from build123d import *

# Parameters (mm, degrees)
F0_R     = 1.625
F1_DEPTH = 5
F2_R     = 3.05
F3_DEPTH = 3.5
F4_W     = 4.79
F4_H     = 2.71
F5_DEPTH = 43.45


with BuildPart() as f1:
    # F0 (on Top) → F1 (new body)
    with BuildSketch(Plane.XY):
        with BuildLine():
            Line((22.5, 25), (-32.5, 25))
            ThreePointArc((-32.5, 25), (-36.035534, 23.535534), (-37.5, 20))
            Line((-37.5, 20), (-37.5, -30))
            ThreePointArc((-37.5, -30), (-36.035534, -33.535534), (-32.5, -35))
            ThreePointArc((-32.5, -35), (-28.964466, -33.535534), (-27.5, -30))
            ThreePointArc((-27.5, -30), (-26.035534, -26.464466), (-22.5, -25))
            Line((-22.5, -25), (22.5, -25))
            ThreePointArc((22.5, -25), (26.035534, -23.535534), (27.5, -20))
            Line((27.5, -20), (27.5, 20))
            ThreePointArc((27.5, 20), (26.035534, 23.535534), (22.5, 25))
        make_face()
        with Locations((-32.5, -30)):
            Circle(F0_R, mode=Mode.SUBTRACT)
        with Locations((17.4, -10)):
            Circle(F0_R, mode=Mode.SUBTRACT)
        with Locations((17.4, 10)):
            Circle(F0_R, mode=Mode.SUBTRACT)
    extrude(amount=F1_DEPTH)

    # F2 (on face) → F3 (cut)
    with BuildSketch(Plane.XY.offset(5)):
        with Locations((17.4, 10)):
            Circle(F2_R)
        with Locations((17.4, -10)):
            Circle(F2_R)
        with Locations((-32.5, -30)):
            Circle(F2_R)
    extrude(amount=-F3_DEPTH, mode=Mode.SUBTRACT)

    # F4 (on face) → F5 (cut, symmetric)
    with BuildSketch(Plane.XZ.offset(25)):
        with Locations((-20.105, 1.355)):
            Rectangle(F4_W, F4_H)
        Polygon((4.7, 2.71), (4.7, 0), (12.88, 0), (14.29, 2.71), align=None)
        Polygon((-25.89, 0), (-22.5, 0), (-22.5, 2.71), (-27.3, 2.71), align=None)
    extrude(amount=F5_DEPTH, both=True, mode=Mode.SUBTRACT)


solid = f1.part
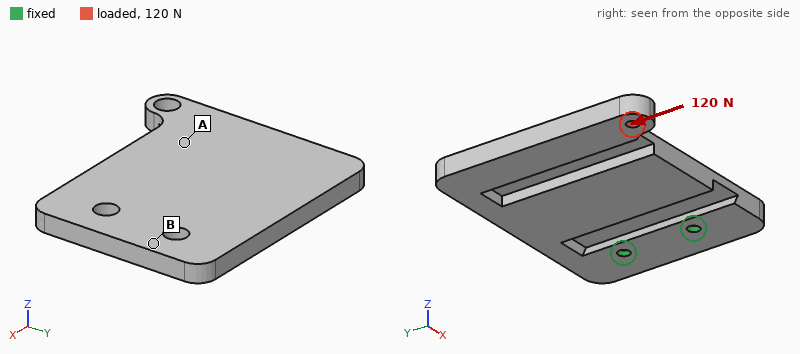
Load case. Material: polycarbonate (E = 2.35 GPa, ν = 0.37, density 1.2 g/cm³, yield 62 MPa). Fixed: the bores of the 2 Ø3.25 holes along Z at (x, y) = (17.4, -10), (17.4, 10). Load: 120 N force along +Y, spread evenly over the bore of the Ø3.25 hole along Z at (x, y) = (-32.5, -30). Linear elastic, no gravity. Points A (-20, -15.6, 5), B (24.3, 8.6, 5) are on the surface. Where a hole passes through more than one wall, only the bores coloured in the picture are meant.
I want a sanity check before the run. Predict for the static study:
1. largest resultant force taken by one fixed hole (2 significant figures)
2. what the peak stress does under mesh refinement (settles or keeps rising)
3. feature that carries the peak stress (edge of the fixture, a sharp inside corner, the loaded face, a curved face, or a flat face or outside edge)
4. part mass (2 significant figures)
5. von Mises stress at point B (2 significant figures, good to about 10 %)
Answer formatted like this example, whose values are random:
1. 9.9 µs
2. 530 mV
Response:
1. 280 N
2. keeps rising
3. edge of the fixture
4. 17 g
5. 6.1 MPa
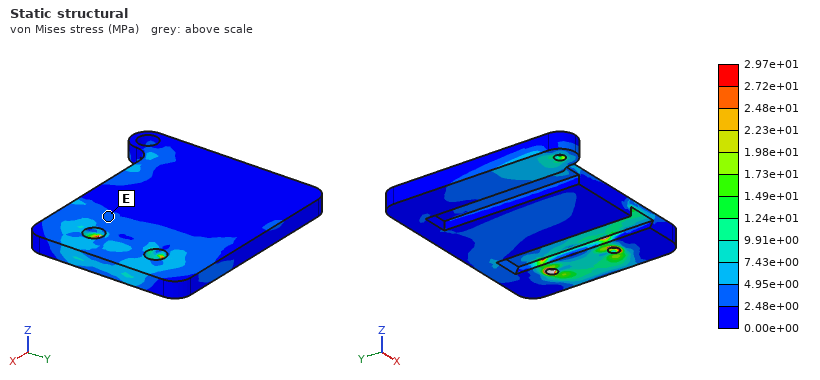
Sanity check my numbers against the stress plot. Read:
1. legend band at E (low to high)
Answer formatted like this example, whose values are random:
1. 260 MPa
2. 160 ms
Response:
1. 2.48e+00 to 4.95e+00 MPa
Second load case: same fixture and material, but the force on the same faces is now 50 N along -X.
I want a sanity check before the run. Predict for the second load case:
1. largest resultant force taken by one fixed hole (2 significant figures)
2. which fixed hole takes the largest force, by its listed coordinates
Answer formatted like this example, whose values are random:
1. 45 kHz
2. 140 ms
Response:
1. 92 N
2. (17.4, -10)
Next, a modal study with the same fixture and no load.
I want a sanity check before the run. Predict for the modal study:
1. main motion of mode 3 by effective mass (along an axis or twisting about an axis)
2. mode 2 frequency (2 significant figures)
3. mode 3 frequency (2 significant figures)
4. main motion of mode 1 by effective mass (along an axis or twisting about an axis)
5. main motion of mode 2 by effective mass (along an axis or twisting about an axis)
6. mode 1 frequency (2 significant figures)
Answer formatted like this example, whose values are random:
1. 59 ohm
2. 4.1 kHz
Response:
1. along Y
2. 570 Hz
3. 920 Hz
4. along Z
5. twisting about X
6. 150 Hz
